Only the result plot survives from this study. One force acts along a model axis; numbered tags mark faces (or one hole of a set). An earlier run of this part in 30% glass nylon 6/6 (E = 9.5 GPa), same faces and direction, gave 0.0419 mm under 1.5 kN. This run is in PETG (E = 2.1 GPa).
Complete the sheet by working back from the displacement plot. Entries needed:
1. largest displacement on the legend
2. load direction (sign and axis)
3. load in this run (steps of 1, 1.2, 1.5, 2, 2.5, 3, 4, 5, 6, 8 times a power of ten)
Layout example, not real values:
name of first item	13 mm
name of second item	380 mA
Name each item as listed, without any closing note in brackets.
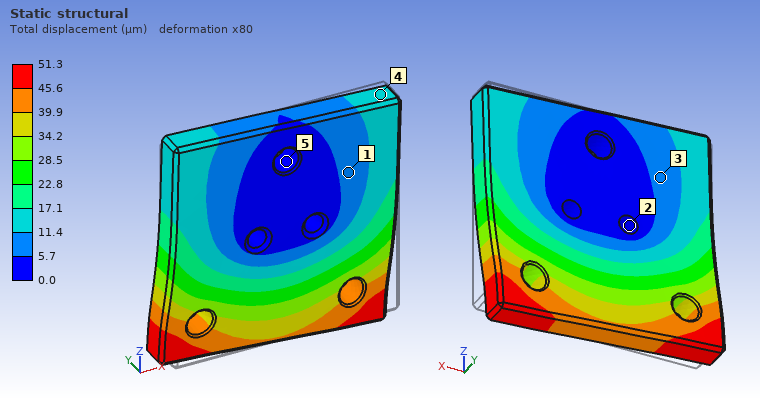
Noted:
largest displacement on the legend	51.3 µm
load direction	-X
load in this run	400 N
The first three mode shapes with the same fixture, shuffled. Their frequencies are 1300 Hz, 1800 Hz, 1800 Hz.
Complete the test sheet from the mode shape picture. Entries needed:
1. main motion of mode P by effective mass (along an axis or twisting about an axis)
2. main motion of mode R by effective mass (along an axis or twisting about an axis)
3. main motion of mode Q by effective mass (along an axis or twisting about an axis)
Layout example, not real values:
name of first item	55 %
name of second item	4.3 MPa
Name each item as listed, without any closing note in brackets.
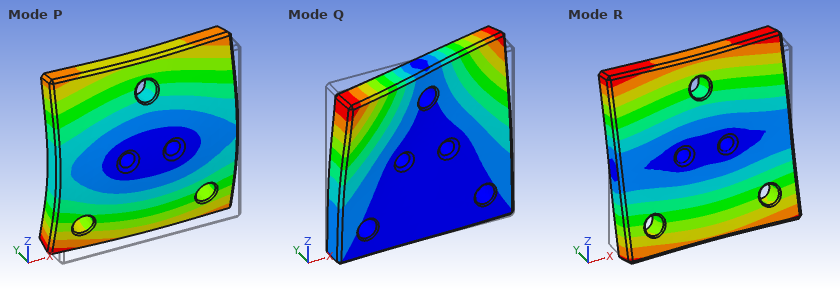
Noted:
main motion of mode P by effective mass	along Y
main motion of mode R by effective mass	twisting about X
main motion of mode Q by effective mass	twisting about Z
